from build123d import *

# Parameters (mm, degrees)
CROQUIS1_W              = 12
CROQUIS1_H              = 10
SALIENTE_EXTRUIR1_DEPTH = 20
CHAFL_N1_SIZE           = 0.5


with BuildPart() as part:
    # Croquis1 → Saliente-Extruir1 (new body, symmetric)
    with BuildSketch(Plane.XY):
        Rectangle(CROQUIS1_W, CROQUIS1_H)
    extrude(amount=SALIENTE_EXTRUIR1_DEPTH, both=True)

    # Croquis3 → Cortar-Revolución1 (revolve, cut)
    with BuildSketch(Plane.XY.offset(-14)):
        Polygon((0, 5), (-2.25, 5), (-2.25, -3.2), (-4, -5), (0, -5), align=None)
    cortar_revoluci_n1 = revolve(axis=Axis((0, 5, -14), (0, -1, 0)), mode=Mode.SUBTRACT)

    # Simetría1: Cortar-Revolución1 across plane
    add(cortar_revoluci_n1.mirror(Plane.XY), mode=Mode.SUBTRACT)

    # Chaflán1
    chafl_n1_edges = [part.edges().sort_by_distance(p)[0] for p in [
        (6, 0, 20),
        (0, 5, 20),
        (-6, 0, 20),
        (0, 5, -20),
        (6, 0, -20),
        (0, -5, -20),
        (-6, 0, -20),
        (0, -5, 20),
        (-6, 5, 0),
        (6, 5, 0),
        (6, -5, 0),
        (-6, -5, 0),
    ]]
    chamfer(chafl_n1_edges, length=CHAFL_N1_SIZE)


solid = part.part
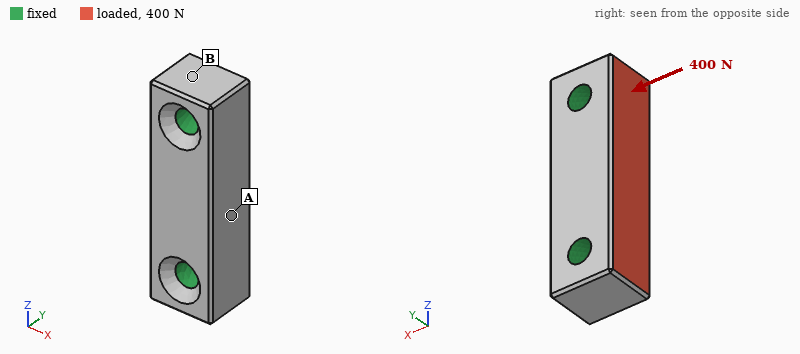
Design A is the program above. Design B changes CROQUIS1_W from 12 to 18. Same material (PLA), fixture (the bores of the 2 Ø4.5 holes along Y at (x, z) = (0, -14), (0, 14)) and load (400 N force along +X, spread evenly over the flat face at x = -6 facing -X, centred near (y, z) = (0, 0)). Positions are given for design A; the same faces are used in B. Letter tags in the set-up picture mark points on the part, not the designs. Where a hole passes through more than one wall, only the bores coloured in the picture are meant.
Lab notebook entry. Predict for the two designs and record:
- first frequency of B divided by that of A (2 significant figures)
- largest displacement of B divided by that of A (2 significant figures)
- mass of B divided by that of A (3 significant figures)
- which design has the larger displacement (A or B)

0.89
0.69
1.55
A
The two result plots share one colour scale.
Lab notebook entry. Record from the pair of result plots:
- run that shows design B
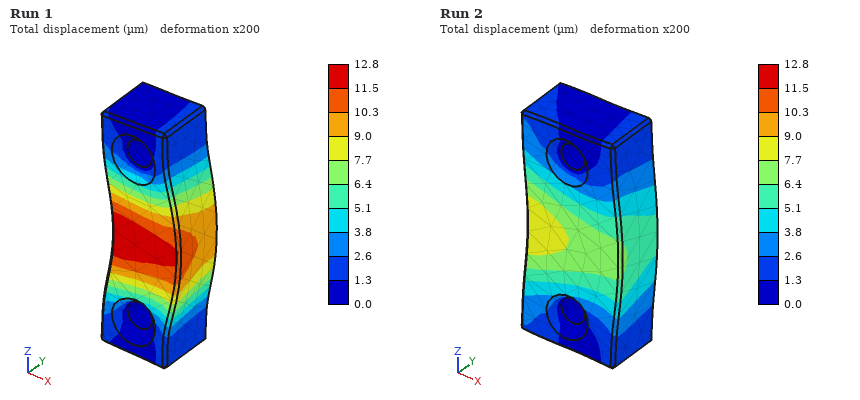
Run 2
